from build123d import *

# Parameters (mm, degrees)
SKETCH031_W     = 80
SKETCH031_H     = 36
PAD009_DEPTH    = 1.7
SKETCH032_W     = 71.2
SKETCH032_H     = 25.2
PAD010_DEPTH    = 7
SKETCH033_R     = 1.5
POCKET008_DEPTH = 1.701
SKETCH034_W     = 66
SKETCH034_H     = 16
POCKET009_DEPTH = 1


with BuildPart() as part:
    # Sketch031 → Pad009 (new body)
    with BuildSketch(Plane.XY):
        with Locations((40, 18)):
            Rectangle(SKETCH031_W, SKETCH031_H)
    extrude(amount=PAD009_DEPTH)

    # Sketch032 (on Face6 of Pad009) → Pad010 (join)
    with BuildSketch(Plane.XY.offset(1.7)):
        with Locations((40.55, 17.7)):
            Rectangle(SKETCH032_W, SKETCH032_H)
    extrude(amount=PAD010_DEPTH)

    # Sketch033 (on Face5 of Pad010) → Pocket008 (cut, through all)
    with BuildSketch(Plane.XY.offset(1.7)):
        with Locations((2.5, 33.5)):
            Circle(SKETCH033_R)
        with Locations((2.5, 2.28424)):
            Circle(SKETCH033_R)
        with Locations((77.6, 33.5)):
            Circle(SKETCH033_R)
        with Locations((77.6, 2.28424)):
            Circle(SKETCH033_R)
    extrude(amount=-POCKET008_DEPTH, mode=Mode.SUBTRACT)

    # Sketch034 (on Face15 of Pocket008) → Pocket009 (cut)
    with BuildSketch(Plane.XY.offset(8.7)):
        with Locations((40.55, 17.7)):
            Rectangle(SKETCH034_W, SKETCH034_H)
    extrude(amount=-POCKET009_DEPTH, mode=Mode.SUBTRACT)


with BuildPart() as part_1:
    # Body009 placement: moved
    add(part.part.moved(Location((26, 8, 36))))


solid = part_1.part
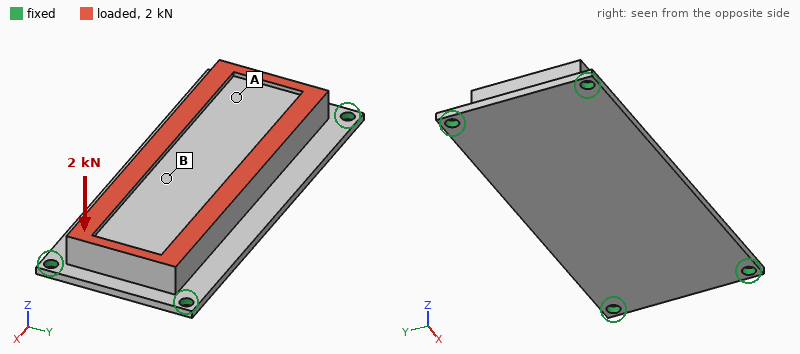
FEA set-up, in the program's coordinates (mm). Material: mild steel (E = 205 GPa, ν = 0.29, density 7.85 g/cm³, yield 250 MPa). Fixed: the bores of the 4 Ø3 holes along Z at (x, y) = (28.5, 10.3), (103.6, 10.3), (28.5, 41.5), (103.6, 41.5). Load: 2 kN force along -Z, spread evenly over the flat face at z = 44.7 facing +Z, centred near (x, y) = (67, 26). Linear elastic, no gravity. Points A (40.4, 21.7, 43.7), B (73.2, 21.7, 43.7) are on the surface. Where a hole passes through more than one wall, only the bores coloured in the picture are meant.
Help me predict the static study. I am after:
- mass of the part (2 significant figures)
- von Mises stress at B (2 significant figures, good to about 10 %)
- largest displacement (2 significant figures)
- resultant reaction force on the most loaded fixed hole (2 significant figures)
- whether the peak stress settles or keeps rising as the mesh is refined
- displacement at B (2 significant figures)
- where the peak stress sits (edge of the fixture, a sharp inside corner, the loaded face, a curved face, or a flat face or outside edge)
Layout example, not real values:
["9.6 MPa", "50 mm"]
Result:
["130 g", "40 MPa", "35 µm", "920 N", "keeps rising", "30 µm", "edge of the fixture"]
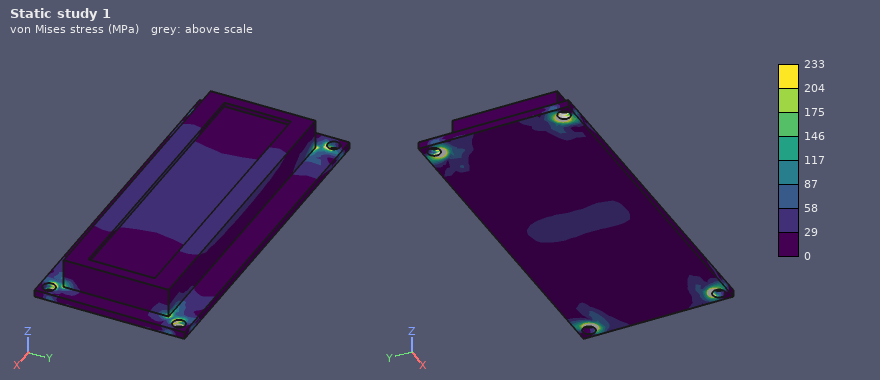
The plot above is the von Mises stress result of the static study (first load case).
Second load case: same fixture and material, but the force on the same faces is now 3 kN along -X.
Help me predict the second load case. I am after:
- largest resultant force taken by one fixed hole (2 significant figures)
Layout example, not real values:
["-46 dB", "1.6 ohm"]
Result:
["830 N"]
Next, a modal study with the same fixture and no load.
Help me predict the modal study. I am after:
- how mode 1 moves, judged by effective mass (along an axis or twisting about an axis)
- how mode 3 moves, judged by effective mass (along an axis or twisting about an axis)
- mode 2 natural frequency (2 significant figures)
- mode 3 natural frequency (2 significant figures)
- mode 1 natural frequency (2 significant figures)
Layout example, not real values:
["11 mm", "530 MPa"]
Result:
["along Z", "twisting about Y", "7600 Hz", "9200 Hz", "3800 Hz"]
